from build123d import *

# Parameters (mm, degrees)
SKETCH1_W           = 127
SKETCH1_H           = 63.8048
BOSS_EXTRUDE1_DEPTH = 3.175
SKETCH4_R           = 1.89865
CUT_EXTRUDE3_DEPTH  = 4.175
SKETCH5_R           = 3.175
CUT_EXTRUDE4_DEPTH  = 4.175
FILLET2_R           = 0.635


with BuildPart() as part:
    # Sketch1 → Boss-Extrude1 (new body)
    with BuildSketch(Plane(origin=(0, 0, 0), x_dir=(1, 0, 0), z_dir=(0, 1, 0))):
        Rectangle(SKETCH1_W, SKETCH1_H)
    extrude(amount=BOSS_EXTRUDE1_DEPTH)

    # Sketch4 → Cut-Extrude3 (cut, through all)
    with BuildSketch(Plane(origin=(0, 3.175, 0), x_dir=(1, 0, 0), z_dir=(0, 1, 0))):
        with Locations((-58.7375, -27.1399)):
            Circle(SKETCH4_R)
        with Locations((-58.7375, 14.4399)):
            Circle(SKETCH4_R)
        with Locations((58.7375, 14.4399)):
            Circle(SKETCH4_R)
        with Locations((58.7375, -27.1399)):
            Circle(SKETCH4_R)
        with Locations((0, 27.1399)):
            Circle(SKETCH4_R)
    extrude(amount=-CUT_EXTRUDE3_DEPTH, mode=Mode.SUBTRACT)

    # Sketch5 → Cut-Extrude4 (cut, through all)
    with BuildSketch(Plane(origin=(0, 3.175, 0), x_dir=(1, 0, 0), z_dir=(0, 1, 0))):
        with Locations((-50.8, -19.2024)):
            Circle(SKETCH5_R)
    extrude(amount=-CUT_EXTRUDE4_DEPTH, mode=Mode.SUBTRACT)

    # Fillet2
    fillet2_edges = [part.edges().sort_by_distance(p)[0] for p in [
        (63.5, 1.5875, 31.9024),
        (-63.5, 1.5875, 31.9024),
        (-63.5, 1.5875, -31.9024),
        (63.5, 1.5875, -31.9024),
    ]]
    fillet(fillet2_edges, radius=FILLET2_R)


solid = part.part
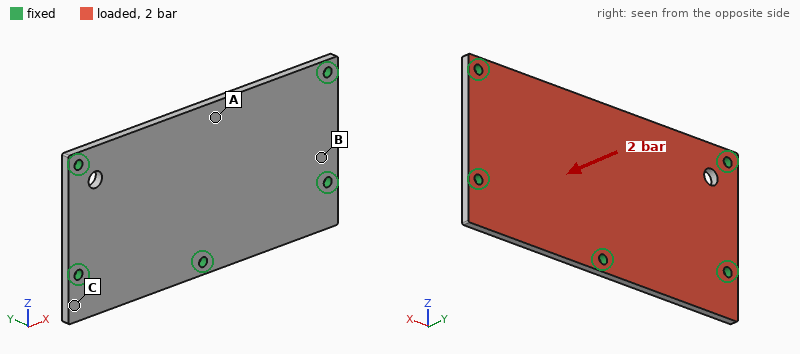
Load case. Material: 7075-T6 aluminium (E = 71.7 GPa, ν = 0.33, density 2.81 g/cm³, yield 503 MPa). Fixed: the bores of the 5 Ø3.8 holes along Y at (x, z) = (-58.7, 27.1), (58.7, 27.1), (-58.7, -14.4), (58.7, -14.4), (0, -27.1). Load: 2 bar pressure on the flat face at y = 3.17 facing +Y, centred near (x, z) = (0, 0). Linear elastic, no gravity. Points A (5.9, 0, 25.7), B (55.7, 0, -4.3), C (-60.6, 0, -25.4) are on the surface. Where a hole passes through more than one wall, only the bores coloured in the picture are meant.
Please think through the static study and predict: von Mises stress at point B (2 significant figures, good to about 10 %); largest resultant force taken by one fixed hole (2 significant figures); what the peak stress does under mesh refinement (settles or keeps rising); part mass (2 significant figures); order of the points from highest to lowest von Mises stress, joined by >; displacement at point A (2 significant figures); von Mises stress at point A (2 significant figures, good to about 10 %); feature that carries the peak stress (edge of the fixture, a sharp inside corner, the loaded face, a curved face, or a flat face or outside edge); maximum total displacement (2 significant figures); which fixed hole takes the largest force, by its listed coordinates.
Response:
29 MPa
540 N
keeps rising
72 g
A > B > C
0.39 mm
44 MPa
edge of the fixture
0.45 mm
(0, -27.1)
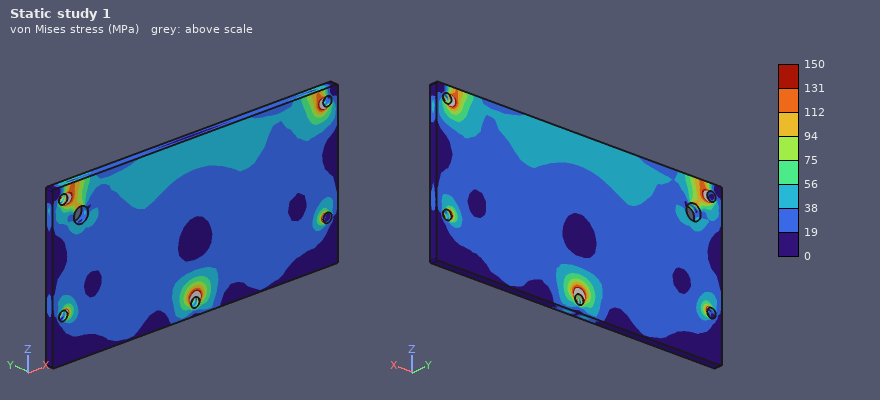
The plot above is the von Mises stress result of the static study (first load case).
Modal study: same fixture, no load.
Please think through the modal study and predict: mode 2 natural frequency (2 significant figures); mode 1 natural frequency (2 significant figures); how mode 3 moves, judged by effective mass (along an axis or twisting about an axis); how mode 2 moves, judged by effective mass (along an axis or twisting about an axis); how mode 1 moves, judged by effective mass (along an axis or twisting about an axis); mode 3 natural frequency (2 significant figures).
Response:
3300 Hz
1500 Hz
along Y
twisting about Z
along Y
4200 Hz
